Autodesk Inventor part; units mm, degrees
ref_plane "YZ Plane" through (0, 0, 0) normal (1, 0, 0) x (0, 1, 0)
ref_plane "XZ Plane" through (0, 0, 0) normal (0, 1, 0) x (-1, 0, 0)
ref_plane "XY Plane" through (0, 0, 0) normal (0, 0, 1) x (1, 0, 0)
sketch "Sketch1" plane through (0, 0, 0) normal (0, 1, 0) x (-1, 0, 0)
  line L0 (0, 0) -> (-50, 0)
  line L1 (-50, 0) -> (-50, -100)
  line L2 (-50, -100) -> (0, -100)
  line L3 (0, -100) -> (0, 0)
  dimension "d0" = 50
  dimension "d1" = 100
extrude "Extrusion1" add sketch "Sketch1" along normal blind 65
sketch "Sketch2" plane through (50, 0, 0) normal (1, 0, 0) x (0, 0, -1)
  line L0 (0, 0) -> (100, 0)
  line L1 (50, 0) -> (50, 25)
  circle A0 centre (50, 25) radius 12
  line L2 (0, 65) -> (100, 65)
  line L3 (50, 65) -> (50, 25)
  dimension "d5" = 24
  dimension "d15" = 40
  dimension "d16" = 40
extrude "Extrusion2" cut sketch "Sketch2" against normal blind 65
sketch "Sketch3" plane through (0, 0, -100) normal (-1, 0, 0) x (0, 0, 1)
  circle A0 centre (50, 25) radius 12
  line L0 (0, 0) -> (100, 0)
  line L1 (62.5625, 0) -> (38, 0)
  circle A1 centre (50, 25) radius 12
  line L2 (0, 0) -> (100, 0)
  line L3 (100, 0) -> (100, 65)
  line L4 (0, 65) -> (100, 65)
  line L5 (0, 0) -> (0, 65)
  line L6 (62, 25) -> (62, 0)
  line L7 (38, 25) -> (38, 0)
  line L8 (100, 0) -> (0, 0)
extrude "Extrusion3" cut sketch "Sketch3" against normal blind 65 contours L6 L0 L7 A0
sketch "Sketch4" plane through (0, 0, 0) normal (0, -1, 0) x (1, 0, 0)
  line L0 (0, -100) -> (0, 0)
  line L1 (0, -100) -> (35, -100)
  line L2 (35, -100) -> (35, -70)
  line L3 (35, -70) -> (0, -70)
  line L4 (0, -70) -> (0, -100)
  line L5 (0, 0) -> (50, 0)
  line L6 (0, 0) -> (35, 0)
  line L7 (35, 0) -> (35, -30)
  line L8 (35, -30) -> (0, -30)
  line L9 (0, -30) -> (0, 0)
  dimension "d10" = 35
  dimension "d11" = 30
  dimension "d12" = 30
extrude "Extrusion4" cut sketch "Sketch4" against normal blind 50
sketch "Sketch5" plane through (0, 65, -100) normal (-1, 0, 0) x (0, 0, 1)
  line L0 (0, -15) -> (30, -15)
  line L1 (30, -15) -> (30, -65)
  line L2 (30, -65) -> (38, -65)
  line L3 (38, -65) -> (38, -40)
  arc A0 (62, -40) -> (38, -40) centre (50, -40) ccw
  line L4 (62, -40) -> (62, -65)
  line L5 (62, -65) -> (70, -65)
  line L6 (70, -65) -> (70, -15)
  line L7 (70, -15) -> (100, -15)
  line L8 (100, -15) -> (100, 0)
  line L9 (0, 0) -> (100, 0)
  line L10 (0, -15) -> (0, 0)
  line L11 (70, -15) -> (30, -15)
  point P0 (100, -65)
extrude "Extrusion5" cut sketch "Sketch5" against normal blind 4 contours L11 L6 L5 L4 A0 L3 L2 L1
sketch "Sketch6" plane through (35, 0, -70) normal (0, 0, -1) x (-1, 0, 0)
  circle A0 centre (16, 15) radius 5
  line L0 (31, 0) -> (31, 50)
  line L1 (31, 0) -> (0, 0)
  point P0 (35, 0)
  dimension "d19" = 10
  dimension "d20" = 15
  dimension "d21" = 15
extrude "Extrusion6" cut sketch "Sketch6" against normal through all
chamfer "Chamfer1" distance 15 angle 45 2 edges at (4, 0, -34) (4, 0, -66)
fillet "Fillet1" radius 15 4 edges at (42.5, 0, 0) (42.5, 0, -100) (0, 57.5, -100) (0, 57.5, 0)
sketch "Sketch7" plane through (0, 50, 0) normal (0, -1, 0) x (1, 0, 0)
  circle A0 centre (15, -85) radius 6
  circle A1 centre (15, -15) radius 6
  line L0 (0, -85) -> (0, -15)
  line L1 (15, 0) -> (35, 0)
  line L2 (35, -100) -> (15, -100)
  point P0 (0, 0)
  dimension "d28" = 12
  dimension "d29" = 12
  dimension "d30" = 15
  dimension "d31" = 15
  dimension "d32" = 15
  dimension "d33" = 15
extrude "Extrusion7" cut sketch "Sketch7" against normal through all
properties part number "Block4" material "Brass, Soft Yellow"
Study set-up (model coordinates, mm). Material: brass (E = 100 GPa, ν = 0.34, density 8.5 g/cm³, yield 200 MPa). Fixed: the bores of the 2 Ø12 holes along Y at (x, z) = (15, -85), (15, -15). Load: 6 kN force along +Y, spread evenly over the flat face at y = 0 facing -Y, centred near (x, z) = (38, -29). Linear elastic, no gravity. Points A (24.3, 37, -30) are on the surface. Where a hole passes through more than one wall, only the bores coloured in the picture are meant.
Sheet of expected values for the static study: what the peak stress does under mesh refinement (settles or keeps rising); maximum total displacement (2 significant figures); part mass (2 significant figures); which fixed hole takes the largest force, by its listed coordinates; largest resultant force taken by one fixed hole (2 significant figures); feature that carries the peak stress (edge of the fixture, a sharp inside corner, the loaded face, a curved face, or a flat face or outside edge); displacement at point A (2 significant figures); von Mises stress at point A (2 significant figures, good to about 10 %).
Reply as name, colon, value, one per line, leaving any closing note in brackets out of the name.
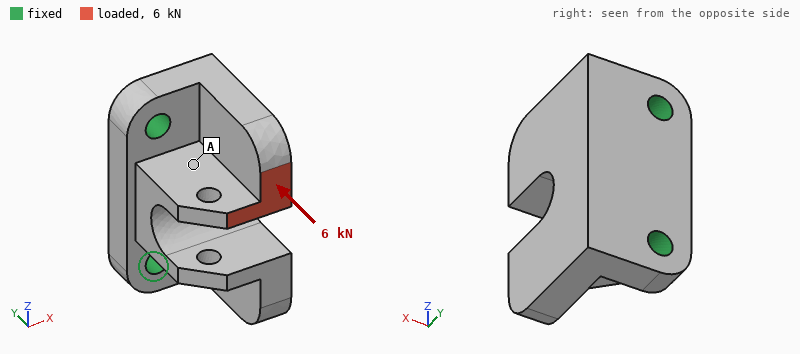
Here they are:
what the peak stress does under mesh refinement: keeps rising
maximum total displacement: 48 µm
part mass: 1.4 kg
which fixed hole takes the largest force, by its listed coordinates: (15, -15)
largest resultant force taken by one fixed hole: 5.0 kN
feature that carries the peak stress: edge of the fixture
displacement at point A: 15 µm
von Mises stress at point A: 8.7 MPa
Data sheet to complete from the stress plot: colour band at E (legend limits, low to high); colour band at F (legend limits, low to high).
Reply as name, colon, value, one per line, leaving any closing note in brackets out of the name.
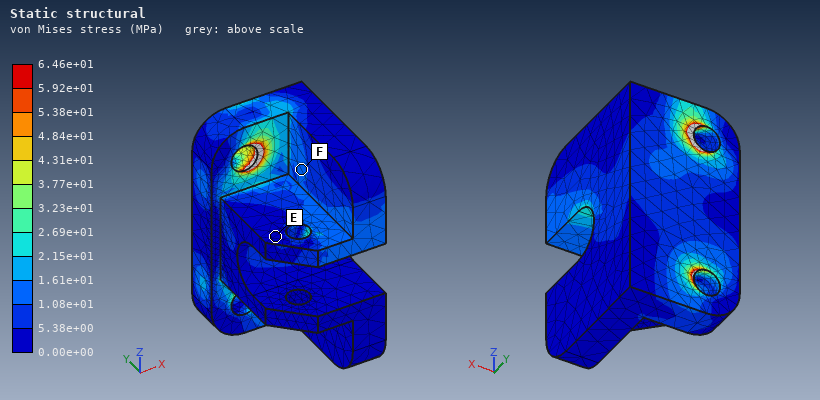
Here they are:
colour band at E: 0.00e+00 to 5.38e+00 MPa
colour band at F: 1.08e+01 to 1.61e+01 MPa
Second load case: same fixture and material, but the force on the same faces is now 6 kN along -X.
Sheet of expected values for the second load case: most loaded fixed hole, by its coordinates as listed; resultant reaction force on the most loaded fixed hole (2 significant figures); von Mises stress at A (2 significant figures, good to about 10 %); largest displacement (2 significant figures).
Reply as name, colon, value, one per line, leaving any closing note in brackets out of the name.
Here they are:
most loaded fixed hole, by its coordinates as listed: (15, -15)
resultant reaction force on the most loaded fixed hole: 4.8 kN
von Mises stress at A: 30 MPa
largest displacement: 0.18 mm
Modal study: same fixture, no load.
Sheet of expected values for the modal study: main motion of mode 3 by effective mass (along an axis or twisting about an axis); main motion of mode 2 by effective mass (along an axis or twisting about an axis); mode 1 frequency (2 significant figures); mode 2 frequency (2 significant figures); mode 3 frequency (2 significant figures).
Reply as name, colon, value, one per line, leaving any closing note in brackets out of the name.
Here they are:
main motion of mode 3 by effective mass: along Z
main motion of mode 2 by effective mass: along Z
mode 1 frequency: 1900 Hz
mode 2 frequency: 3700 Hz
mode 3 frequency: 4400 Hz
